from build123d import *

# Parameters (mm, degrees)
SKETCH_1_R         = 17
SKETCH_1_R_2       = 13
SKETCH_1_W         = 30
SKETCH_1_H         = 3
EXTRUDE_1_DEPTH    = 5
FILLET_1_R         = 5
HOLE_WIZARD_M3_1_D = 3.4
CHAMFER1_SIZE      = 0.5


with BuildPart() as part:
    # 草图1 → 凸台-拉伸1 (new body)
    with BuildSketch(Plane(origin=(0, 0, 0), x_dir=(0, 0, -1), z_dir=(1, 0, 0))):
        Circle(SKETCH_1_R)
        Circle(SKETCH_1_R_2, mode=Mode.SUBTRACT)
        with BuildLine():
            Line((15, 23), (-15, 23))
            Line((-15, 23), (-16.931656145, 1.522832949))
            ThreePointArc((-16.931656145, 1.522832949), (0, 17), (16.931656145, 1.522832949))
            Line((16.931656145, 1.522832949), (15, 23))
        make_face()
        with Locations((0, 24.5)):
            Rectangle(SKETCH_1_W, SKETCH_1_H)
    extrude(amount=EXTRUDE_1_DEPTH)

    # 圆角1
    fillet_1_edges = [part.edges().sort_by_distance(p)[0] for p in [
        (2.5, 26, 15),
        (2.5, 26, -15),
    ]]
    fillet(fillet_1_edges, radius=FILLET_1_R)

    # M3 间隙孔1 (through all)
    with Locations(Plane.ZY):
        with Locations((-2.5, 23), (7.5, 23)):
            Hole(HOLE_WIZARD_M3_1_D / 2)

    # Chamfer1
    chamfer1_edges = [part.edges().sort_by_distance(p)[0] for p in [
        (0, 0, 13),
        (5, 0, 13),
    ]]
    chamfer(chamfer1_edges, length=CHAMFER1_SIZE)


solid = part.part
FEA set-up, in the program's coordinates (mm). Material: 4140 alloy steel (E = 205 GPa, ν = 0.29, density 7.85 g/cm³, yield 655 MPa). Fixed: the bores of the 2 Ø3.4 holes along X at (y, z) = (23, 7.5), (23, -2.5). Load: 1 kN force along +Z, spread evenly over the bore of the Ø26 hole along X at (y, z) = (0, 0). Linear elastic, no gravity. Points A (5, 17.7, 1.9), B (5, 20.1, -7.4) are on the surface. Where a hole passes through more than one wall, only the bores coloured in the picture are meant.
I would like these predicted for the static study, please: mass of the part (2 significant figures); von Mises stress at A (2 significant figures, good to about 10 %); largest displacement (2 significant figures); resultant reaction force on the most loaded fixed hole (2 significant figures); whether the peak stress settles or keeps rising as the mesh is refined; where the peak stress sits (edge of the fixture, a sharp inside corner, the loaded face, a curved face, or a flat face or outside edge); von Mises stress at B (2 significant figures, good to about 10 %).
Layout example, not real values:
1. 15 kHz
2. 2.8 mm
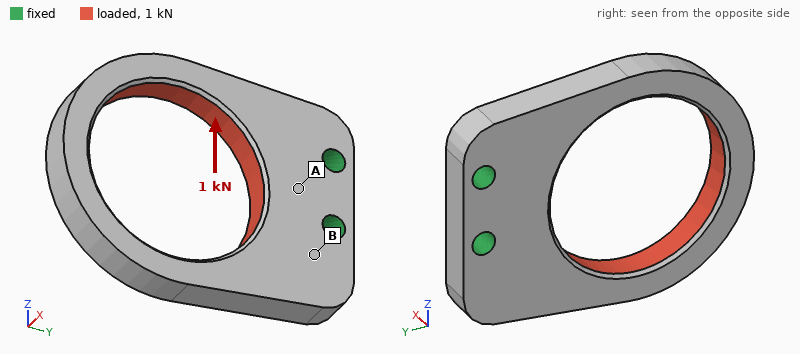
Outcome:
1. 28 g
2. 65 MPa
3. 59 µm
4. 1.6 kN
5. keeps rising
6. edge of the fixture
7. 23 MPa
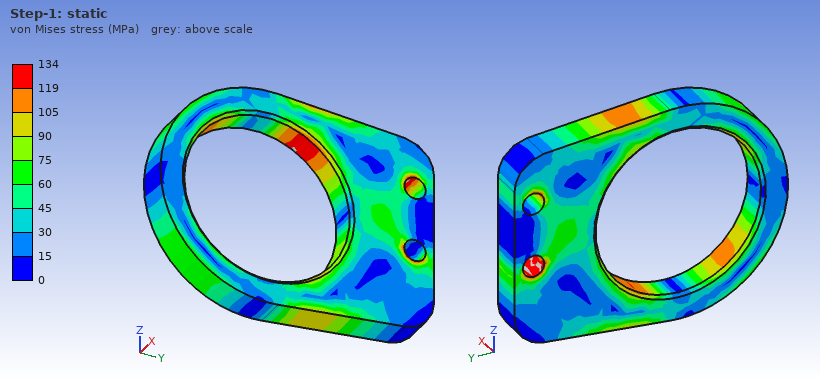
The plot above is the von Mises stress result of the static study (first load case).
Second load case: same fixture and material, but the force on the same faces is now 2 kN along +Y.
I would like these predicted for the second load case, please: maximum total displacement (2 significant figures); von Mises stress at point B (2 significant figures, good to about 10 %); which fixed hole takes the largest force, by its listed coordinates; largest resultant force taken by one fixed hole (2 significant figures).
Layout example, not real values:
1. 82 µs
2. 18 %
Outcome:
1. 21 µm
2. 40 MPa
3. (23, -2.5)
4. 1.5 kN
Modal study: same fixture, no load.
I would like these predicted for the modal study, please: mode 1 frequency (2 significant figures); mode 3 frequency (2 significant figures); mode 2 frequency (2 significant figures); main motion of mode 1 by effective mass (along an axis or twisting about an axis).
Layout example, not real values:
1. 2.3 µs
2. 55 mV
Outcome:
1. 2900 Hz
2. 6200 Hz
3. 5900 Hz
4. along X
